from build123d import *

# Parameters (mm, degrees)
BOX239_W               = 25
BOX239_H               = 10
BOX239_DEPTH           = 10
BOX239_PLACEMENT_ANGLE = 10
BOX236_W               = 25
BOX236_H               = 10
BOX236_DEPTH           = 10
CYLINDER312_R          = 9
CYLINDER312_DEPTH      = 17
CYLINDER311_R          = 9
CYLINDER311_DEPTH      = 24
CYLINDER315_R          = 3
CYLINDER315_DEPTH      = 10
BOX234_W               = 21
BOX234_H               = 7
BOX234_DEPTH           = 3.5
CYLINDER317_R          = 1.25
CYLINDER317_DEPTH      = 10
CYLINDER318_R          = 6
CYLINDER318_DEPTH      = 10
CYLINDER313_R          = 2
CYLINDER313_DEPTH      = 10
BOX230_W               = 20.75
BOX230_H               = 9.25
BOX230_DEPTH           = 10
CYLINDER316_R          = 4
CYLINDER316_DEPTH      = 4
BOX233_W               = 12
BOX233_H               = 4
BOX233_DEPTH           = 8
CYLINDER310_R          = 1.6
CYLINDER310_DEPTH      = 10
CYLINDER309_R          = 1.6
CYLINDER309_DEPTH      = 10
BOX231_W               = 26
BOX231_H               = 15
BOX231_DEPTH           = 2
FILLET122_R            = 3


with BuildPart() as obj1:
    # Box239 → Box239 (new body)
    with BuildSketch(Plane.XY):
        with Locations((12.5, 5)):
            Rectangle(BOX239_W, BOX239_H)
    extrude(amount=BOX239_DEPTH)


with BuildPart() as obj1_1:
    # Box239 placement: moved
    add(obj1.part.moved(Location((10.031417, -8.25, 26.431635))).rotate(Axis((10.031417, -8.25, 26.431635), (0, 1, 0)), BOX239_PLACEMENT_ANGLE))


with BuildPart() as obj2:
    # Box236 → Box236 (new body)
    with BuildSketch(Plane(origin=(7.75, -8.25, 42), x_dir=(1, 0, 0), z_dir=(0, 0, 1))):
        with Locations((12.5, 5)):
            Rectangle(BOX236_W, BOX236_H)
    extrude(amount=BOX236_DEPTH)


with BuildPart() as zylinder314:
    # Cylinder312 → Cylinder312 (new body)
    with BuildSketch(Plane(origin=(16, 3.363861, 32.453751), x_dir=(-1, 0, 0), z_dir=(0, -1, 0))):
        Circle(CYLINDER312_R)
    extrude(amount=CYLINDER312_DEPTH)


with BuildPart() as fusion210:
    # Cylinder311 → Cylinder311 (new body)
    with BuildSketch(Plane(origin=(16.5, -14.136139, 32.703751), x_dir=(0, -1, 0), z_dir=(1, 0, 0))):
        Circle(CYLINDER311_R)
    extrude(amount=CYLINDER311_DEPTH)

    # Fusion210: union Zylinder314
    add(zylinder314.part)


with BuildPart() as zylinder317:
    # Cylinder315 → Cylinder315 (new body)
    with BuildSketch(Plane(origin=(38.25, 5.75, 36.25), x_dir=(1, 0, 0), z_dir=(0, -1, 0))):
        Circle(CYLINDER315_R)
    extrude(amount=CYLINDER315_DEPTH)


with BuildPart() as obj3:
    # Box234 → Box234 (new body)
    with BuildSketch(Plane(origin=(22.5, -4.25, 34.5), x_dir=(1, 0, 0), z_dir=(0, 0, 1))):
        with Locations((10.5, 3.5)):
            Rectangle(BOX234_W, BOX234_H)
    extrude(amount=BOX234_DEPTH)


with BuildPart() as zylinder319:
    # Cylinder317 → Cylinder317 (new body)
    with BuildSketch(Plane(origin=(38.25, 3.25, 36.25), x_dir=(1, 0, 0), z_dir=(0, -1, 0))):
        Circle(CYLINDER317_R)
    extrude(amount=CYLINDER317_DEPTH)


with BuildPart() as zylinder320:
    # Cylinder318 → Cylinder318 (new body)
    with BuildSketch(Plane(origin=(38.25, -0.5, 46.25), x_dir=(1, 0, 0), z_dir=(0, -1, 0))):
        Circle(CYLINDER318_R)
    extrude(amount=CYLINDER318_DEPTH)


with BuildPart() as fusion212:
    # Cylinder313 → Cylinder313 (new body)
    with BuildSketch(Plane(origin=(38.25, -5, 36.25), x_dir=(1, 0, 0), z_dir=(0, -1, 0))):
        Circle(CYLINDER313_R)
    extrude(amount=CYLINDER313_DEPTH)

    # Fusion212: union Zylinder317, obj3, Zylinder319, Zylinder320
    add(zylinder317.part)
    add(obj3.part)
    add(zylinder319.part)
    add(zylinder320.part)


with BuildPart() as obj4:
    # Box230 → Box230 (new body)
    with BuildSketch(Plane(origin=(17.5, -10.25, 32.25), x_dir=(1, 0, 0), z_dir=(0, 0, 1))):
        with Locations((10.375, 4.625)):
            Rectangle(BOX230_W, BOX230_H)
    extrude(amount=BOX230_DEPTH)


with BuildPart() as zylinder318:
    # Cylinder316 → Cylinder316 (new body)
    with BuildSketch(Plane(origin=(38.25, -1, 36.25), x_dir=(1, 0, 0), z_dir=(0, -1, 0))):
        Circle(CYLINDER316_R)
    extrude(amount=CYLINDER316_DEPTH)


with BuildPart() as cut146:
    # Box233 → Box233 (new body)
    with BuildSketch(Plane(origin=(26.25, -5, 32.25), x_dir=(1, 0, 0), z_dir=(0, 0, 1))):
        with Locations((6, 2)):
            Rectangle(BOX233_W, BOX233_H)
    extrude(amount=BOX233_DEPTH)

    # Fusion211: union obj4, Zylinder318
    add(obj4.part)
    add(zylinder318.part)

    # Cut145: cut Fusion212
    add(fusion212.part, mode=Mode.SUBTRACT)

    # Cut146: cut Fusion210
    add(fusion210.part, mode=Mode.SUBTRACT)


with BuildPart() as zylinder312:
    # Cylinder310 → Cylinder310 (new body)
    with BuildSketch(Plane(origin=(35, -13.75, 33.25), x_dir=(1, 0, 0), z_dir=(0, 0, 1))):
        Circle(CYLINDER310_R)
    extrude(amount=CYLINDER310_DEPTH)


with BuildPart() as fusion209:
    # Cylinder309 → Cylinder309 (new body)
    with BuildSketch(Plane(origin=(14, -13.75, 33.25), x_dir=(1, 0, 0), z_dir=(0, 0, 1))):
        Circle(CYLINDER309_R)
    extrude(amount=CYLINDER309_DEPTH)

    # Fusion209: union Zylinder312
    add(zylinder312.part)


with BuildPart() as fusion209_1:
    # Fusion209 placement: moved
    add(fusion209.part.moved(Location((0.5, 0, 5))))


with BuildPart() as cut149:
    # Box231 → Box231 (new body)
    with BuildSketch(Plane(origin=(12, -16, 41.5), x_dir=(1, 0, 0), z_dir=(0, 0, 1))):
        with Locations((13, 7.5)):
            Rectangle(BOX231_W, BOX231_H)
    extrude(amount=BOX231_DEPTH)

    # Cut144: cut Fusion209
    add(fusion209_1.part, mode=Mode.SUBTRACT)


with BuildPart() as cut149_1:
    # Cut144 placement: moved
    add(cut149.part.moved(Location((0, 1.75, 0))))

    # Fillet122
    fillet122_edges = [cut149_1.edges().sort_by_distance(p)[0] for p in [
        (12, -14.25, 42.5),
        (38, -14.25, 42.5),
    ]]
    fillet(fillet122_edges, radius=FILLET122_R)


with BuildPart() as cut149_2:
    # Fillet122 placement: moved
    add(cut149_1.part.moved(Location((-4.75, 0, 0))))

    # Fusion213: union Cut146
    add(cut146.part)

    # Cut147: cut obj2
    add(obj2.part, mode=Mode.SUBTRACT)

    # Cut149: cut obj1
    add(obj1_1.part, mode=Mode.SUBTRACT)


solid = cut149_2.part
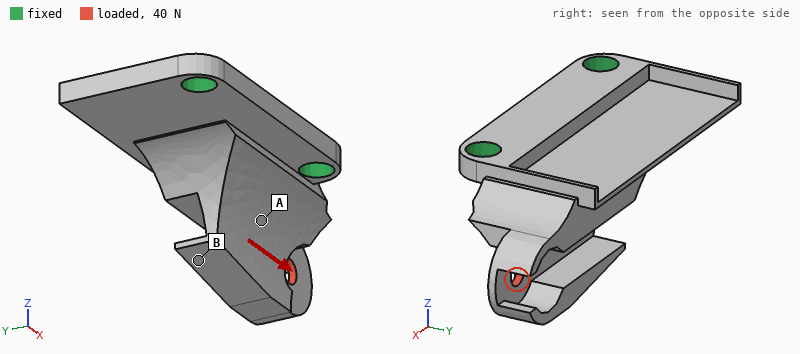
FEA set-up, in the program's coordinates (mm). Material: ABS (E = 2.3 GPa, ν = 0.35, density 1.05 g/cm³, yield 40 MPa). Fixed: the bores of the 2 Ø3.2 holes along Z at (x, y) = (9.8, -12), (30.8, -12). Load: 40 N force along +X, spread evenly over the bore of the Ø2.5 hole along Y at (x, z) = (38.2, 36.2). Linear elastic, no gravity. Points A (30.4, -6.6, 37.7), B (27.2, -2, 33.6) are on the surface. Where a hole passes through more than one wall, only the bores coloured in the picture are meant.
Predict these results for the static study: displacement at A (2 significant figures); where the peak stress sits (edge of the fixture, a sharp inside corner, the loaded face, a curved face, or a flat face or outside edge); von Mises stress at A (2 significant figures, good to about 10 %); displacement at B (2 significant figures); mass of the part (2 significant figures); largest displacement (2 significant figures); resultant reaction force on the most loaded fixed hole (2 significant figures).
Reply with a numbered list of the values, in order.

1. 0.049 mm
2. edge of the fixture
3. 4.2 MPa
4. 0.095 mm
5. 1.1 g
6. 0.17 mm
7. 25 N
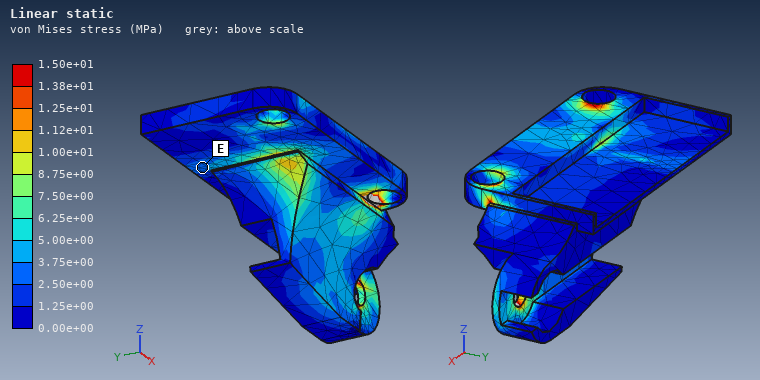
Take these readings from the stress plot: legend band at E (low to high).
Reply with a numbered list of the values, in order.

1. 2.50e+00 to 3.75e+00 MPa
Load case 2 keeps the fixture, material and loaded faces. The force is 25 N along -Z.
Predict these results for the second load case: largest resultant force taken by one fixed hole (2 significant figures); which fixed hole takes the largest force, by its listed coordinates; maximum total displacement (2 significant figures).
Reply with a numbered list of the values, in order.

1. 32 N
2. (30.8, -12)
3. 0.48 mm
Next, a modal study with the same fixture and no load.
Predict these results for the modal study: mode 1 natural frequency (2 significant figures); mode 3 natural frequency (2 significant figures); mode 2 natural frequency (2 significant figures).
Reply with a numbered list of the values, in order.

1. 1900 Hz
2. 4000 Hz
3. 3400 Hz
